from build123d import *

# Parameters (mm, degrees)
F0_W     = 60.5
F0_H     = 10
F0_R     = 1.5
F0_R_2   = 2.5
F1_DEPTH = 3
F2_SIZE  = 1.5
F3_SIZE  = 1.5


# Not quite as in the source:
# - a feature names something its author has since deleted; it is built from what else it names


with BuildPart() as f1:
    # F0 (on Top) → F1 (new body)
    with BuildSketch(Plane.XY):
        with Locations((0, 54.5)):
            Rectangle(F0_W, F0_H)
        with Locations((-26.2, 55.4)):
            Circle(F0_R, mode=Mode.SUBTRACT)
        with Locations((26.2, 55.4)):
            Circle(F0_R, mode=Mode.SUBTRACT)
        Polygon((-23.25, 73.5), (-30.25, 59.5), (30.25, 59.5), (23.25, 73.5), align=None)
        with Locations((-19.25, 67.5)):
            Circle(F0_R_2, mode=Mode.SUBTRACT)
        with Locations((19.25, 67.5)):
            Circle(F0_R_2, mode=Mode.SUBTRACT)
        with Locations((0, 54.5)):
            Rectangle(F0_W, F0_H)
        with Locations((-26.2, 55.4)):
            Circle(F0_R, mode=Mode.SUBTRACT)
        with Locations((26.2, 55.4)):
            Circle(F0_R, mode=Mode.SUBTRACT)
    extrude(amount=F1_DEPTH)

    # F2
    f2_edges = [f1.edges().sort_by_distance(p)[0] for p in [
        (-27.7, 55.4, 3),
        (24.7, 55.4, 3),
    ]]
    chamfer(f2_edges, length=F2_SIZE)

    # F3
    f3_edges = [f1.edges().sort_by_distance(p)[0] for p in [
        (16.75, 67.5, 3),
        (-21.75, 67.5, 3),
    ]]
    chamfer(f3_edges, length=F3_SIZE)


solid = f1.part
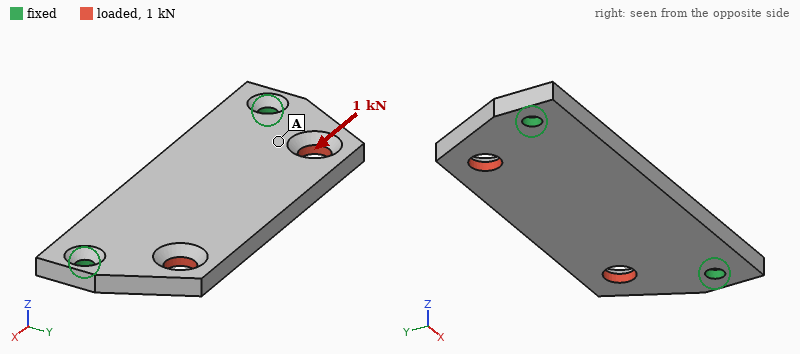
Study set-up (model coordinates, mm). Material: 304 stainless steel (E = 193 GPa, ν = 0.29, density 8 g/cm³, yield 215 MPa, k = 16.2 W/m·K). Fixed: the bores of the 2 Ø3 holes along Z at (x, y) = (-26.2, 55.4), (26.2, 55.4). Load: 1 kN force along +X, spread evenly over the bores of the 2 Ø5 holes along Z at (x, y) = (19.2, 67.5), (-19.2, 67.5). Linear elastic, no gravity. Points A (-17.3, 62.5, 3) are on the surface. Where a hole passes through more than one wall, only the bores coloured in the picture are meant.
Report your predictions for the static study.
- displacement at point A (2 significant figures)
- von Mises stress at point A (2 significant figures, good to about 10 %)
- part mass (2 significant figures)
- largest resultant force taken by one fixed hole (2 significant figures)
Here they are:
1.6 µm
9.3 MPa
31 g
550 N
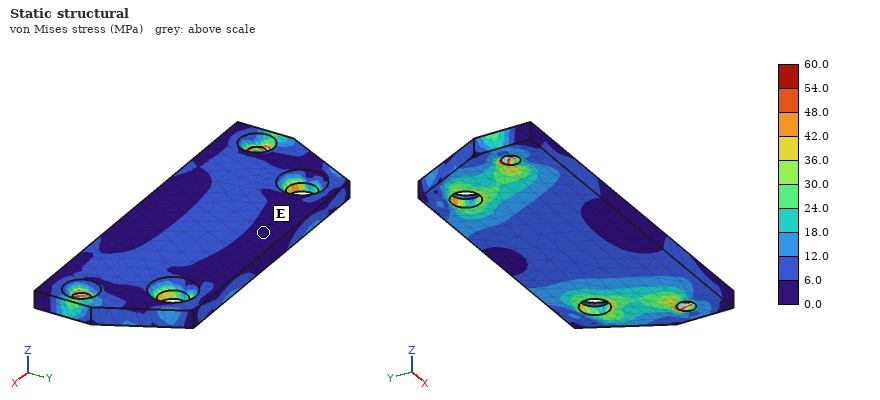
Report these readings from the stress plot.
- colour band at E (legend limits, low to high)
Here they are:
0.0 to 6.0 MPa
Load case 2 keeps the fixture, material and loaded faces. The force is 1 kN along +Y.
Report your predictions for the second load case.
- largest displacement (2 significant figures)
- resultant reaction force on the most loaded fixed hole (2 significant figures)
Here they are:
7.9 µm
530 N
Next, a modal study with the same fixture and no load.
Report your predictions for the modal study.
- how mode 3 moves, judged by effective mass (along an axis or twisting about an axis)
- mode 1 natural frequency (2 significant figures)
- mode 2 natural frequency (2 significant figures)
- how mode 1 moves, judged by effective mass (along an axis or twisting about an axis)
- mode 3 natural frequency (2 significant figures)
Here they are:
twisting about Y
3100 Hz
5800 Hz
along Z
7900 Hz
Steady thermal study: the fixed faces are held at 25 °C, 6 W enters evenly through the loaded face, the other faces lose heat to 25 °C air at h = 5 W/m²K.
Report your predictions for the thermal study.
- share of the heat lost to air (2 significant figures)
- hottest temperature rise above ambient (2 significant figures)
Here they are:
9.8 %
73 K
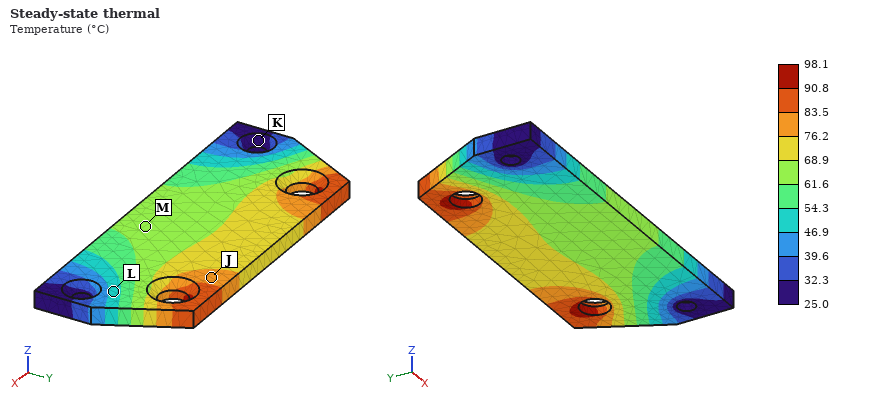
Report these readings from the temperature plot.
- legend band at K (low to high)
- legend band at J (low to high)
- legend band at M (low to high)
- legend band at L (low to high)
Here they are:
25.0 to 32.3 °C
76.2 to 83.5 °C
61.6 to 68.9 °C
46.9 to 54.3 °C
